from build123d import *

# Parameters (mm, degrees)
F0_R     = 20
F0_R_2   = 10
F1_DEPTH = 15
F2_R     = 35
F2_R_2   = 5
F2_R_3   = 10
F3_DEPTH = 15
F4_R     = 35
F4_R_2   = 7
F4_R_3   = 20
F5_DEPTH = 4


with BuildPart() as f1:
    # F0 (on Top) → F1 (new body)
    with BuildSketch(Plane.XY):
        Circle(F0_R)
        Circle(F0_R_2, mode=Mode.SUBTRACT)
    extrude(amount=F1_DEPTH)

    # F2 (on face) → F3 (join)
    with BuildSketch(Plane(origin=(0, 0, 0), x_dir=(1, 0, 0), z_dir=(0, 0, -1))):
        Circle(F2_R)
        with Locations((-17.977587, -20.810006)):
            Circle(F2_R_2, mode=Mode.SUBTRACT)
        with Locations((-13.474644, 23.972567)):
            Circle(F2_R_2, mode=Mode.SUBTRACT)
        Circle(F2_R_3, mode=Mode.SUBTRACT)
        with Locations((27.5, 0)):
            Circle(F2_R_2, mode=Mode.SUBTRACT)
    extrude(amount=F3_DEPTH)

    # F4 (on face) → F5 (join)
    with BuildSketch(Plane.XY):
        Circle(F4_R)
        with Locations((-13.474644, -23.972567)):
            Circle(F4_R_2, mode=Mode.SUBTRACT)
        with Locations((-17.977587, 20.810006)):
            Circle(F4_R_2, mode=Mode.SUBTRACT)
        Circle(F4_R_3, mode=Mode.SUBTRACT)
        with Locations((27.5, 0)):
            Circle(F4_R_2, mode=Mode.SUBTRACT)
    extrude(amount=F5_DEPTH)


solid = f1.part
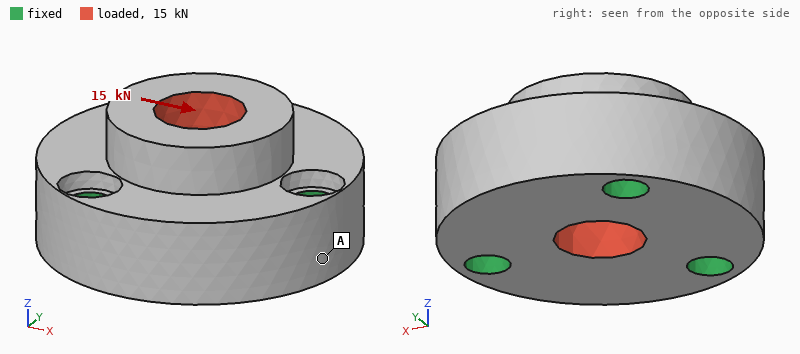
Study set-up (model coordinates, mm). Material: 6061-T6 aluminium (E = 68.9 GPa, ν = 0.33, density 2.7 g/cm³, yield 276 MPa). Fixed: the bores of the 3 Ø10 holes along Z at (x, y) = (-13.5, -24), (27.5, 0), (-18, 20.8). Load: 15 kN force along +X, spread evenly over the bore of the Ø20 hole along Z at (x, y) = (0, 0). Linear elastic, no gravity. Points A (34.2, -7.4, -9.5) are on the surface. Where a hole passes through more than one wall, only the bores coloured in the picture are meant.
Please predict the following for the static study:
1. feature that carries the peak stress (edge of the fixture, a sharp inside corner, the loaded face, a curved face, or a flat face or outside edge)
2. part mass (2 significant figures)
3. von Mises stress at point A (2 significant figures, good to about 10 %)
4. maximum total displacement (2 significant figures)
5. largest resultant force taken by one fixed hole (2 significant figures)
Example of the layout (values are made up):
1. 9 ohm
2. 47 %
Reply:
1. edge of the fixture
2. 190 g
3. 5.6 MPa
4. 11 µm
5. 5.6 kN
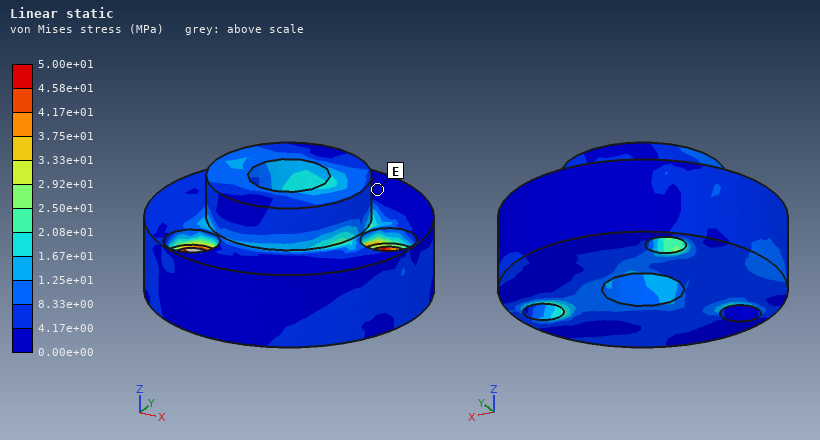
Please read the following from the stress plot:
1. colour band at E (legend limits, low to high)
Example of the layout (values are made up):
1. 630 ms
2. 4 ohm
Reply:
1. 0.00e+00 to 4.17e+00 MPa
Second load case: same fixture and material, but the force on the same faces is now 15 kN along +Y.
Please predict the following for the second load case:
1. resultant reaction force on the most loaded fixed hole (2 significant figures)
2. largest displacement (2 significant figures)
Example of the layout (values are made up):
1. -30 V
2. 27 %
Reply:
1. 5.4 kN
2. 12 µm
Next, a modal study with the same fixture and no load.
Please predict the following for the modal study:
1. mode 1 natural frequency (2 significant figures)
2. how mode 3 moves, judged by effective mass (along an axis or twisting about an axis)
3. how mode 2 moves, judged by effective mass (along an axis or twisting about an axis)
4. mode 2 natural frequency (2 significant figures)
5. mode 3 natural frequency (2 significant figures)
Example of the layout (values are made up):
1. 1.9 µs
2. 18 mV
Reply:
1. 16 kHz
2. along Z
3. along Z
4. 19 kHz
5. 22 kHz
